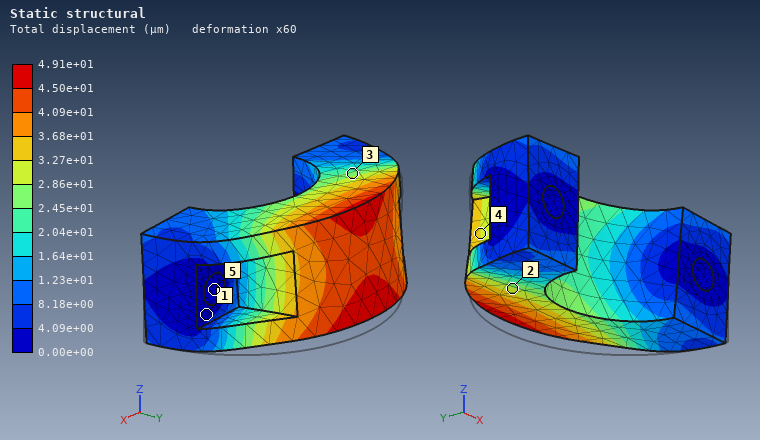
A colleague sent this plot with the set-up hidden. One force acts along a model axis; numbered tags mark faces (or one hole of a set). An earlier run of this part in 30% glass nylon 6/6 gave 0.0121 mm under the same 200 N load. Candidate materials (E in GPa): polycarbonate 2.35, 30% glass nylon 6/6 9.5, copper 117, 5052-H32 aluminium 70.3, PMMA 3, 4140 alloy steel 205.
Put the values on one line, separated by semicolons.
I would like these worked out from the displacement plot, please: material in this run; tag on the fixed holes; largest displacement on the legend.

polycarbonate; 5; 4.91e+01 µm
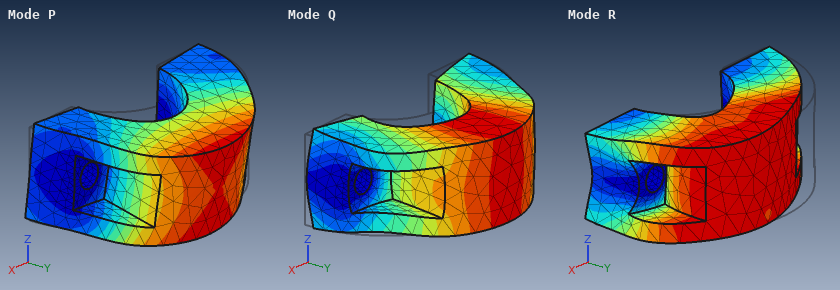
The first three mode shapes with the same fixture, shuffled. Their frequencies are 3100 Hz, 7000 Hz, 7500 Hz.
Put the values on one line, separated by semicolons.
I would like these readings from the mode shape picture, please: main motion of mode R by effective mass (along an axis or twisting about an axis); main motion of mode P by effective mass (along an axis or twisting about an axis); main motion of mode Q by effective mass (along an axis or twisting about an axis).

along X; along Z; along Y
